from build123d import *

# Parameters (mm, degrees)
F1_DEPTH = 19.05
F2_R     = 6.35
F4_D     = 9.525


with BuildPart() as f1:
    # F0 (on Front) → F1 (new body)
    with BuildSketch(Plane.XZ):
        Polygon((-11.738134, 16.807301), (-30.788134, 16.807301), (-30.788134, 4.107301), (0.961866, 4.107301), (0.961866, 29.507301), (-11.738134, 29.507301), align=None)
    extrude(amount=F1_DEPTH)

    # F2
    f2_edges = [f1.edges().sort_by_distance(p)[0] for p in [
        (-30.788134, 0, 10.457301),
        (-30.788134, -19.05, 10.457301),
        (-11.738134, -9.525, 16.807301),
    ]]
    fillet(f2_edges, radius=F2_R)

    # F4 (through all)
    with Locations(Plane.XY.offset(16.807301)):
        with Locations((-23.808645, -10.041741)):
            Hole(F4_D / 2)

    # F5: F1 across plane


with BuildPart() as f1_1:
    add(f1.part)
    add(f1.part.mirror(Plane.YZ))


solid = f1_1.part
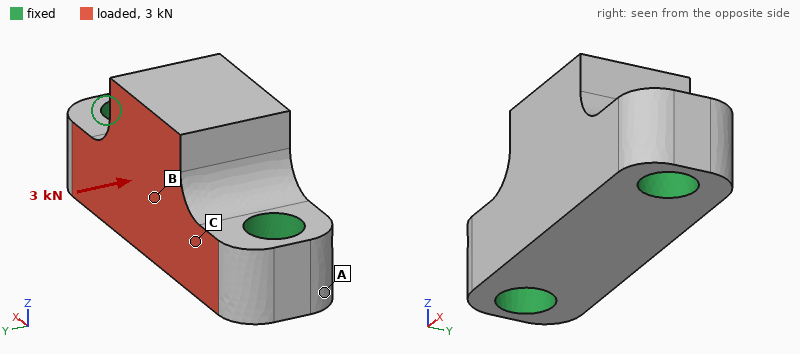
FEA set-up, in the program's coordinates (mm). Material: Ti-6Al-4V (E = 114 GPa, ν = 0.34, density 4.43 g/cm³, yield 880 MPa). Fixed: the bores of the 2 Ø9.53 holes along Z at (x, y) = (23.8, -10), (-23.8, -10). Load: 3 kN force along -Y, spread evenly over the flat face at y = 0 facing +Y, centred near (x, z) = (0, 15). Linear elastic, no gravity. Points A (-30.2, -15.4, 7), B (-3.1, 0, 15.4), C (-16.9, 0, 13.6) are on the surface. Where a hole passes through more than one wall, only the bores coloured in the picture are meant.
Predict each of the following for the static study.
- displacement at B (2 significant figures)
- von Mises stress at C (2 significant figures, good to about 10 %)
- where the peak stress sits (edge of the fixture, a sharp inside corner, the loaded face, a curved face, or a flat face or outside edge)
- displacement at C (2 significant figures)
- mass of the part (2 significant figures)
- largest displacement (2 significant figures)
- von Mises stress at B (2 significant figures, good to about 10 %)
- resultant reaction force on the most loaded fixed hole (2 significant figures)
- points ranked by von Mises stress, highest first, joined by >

3.9 µm
14 MPa
edge of the fixture
1.8 µm
83 g
7.0 µm
8.3 MPa
1.5 kN
C > B > A
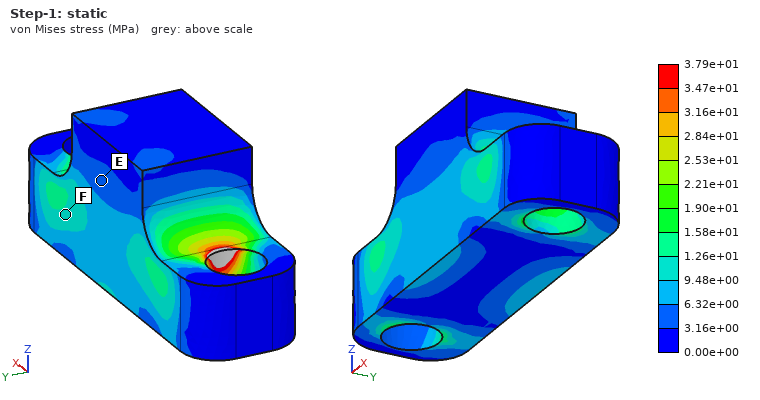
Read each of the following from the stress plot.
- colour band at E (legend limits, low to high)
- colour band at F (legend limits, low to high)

3.16e+00 to 6.32e+00 MPa
9.48e+00 to 1.26e+01 MPa
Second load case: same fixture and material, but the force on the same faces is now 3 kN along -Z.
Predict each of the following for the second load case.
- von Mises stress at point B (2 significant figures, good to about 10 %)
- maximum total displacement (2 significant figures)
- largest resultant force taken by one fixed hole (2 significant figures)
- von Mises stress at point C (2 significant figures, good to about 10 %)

6.7 MPa
9.6 µm
1.5 kN
30 MPa
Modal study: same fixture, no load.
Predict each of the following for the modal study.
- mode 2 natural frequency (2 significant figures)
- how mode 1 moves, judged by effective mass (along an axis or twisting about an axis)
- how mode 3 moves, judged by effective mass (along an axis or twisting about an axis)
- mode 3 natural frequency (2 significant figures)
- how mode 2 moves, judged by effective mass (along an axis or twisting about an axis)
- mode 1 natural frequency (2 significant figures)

23 kHz
along Y
along Y
27 kHz
along Z
14 kHz
